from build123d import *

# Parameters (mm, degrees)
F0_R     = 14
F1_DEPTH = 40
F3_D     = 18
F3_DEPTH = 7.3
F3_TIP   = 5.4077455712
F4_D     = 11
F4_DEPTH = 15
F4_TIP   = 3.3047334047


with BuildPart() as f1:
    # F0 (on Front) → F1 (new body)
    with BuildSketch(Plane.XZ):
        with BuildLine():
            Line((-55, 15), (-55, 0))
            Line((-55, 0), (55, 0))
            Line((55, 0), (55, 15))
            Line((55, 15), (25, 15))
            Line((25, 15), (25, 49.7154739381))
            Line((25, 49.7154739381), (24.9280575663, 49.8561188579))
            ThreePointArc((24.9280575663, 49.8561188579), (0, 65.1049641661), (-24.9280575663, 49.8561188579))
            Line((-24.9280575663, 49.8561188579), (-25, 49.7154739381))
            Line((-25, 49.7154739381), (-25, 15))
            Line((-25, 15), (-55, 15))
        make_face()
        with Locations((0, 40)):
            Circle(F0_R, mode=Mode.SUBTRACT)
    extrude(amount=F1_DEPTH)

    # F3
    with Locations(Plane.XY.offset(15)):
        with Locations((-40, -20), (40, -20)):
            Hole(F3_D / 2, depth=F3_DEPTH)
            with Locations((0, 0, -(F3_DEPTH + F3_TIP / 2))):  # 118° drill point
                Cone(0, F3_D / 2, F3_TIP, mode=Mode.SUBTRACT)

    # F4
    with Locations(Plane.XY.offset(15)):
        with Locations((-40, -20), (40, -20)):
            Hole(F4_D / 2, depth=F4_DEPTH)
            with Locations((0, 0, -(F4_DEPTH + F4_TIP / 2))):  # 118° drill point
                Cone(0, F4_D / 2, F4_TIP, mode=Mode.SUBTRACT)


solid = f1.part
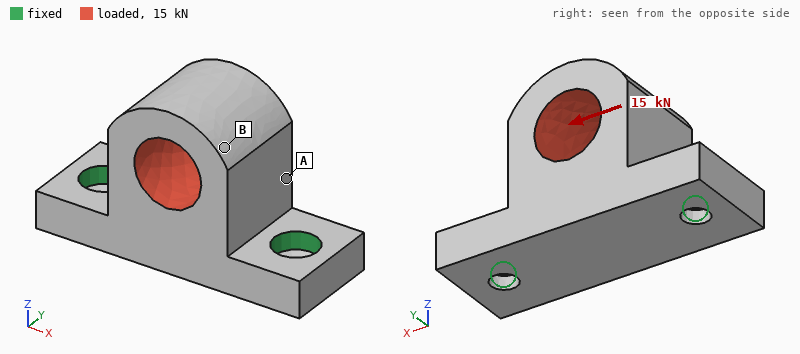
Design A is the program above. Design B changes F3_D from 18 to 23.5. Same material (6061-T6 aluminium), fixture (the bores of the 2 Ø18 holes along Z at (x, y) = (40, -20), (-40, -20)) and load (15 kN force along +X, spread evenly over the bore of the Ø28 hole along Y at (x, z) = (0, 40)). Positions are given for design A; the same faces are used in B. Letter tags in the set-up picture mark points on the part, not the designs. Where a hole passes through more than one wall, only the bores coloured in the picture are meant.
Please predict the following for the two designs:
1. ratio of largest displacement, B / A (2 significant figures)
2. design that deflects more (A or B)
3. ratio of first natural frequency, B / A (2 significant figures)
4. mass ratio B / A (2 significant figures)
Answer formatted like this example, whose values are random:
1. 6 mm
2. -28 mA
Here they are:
1. 0.88
2. A
3. 1.2
4. 0.98
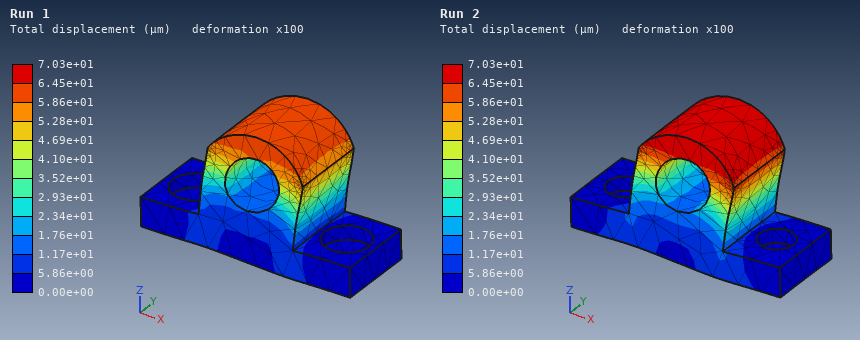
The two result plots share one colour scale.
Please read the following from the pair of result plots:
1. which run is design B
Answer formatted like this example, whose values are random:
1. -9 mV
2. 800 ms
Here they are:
1. Run 1
